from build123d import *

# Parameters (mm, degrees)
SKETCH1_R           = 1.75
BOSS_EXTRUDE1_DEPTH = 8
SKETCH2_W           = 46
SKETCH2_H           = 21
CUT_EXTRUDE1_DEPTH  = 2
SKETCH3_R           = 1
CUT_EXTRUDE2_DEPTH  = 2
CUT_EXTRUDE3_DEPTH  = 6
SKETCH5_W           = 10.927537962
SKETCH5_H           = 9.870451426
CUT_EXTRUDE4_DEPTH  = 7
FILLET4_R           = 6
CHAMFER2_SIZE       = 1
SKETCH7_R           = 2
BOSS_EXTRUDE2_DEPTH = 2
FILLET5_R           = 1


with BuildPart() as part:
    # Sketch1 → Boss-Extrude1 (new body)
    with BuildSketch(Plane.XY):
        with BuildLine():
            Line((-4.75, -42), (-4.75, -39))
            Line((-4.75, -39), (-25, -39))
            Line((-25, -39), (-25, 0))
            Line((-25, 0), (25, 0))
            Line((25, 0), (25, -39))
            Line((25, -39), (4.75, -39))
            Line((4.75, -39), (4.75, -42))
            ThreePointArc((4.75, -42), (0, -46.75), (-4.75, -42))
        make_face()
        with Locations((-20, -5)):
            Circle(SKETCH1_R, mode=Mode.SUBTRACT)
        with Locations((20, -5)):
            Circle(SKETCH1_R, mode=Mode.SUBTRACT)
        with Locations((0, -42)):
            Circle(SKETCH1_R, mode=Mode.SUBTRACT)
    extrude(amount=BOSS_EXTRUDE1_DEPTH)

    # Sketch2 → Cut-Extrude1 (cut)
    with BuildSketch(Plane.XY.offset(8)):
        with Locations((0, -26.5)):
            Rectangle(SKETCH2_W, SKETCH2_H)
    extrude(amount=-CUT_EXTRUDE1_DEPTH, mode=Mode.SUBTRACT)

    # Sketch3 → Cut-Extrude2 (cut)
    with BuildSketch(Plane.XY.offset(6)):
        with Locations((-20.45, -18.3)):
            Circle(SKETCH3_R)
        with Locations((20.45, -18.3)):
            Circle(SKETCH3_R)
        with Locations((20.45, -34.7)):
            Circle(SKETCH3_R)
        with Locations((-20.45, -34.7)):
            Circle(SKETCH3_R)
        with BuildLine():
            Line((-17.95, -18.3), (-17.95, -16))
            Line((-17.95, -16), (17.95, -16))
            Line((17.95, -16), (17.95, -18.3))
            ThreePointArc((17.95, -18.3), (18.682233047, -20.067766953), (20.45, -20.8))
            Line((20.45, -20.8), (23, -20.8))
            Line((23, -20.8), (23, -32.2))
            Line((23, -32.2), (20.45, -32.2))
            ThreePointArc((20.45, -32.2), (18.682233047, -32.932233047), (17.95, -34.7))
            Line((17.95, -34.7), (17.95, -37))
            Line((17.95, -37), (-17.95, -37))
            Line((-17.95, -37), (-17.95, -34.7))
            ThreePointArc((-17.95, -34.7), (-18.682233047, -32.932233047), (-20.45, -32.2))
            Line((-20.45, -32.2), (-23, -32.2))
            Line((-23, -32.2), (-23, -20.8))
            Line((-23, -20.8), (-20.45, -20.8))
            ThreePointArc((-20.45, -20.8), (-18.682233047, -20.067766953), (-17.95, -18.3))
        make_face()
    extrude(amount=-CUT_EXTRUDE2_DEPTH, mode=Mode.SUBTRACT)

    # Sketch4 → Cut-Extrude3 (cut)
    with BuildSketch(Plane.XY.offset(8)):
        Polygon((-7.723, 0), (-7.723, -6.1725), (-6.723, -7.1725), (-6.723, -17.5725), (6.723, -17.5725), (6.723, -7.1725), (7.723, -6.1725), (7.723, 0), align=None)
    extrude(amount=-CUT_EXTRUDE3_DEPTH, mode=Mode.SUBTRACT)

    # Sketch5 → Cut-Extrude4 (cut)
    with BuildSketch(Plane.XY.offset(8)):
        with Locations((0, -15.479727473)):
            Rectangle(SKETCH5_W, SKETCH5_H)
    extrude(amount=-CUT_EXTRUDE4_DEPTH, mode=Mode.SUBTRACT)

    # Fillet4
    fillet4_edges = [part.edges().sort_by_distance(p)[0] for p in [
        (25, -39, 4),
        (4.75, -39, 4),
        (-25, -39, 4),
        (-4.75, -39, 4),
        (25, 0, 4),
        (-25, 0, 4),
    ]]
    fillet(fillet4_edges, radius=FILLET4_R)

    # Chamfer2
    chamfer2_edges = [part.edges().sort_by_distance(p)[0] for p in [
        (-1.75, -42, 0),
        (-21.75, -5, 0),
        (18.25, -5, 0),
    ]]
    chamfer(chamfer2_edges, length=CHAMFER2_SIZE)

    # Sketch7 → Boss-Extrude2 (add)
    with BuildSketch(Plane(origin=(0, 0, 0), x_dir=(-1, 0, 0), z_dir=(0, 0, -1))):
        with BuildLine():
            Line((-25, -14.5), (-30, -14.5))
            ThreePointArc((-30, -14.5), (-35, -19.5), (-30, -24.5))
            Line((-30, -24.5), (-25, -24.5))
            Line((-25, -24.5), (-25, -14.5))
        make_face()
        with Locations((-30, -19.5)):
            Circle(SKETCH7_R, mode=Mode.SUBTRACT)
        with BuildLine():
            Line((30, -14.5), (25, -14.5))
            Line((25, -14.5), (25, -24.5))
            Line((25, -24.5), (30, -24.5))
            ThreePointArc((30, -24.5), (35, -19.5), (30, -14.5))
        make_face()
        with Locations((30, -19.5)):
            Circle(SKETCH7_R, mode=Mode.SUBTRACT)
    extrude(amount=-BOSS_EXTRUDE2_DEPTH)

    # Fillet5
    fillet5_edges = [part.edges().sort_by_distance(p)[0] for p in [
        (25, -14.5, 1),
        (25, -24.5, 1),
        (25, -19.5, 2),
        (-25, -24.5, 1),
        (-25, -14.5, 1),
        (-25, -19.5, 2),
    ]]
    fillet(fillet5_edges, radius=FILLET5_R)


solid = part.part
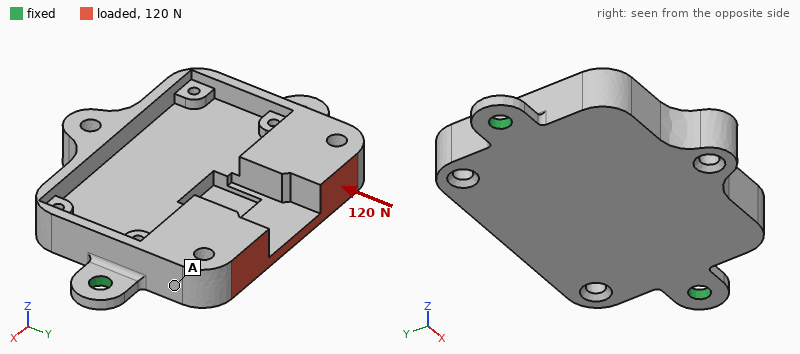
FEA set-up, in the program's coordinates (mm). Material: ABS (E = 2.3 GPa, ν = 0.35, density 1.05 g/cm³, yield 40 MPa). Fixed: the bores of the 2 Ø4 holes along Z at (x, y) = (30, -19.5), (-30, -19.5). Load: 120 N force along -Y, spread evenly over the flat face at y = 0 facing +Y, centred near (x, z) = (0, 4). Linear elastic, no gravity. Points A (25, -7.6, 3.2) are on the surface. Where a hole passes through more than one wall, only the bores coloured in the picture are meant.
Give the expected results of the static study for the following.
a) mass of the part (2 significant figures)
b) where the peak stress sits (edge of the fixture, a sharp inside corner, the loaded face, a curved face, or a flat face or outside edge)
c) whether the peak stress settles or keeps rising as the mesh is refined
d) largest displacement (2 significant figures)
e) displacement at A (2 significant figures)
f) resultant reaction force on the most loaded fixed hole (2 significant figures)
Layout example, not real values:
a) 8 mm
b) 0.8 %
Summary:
a) 11 g
b) edge of the fixture
c) keeps rising
d) 0.52 mm
e) 0.22 mm
f) 60 N
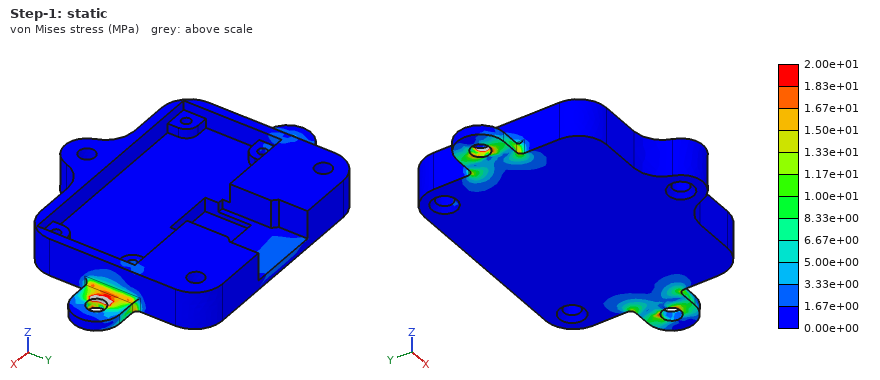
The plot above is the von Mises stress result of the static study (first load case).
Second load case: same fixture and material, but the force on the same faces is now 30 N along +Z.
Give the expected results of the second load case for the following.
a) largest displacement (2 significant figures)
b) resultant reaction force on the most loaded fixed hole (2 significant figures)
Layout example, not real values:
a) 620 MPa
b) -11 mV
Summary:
a) 0.97 mm
b) 21 N
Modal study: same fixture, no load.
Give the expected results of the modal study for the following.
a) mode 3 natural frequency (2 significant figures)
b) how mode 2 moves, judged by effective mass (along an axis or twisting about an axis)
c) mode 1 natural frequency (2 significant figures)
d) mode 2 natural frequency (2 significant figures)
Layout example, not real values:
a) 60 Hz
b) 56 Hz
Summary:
a) 1600 Hz
b) along Z
c) 480 Hz
d) 840 Hz
